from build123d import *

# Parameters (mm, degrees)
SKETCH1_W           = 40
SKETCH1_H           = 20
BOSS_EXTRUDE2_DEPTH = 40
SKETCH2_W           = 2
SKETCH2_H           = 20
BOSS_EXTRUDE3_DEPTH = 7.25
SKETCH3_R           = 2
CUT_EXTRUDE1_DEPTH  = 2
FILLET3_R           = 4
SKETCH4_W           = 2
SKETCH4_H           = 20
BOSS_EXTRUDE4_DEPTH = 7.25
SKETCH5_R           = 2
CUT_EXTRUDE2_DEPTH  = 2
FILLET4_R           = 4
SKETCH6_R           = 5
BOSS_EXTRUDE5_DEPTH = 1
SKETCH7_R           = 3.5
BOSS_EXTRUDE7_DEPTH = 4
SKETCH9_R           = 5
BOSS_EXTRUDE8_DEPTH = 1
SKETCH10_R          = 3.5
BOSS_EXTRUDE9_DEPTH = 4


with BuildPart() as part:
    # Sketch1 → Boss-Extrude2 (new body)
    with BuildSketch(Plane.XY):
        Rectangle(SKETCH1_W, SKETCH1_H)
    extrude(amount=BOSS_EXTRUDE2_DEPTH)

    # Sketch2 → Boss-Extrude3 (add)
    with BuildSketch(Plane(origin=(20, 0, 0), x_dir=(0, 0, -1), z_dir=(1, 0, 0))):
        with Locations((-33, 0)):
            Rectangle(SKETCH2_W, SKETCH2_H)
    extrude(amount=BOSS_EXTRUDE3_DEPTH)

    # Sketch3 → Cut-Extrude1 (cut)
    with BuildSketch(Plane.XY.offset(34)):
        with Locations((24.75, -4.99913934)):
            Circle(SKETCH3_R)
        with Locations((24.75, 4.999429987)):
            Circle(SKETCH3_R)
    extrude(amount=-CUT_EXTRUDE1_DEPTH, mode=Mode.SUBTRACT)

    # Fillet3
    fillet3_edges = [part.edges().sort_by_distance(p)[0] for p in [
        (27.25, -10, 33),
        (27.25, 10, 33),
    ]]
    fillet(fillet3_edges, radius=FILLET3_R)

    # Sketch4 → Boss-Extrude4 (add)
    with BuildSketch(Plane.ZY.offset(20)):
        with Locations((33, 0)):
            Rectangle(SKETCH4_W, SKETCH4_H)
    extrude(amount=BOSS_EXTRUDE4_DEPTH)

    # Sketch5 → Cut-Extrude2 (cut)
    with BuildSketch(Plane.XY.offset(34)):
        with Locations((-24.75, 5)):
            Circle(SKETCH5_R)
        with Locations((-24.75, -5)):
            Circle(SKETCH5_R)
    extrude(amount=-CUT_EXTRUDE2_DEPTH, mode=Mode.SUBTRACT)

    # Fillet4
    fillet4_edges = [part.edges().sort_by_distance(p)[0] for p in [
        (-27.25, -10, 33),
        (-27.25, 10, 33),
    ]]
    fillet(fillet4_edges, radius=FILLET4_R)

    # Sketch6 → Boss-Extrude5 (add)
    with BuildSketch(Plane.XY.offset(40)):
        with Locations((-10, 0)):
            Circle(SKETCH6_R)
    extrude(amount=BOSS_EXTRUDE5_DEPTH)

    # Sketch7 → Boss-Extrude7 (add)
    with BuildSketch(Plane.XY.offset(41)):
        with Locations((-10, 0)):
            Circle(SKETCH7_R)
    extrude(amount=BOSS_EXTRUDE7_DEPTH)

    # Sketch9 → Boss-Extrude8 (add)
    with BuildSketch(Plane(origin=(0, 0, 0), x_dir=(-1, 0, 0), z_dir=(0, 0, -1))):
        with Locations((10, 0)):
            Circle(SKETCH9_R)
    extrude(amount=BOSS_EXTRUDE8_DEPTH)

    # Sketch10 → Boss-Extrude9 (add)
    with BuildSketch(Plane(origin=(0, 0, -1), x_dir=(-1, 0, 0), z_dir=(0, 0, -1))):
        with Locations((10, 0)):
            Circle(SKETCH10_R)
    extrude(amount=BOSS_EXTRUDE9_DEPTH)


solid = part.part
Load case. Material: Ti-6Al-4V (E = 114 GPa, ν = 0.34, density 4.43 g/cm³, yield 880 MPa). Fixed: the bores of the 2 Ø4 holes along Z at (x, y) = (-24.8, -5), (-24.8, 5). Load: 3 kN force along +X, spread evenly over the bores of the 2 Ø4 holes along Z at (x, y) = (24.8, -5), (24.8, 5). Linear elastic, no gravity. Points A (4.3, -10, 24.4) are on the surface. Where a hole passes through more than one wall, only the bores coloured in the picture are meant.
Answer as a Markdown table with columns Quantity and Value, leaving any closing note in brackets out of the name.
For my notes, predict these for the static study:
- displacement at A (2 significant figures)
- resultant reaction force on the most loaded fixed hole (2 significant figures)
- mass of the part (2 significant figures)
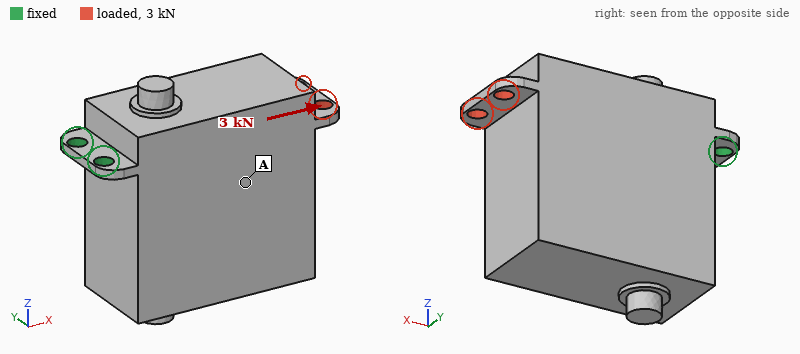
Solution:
| Quantity | Value |
|---|---|
| displacement at A | 5.4 µm |
| resultant reaction force on the most loaded fixed hole | 1.5 kN |
| mass of the part | 150 g |
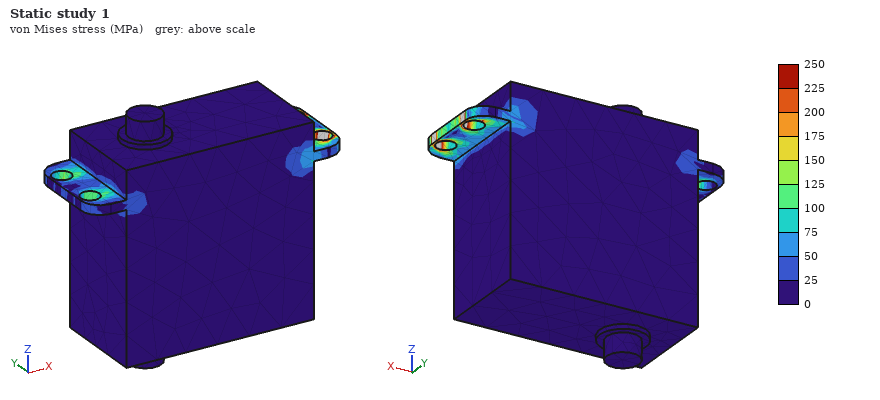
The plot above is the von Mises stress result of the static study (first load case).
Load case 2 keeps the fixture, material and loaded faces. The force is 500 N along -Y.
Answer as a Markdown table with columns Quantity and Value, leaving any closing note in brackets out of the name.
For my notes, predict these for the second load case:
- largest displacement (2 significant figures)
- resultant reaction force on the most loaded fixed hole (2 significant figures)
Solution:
| Quantity | Value |
|---|---|
| largest displacement | 73 µm |
| resultant reaction force on the most loaded fixed hole | 2.0 kN |
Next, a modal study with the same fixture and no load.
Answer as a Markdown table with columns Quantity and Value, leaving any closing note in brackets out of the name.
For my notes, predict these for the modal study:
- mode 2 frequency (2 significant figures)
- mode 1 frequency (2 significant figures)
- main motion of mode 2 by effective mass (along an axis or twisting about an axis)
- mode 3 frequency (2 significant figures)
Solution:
| Quantity | Value |
|---|---|
| mode 2 frequency | 1400 Hz |
| mode 1 frequency | 280 Hz |
| main motion of mode 2 by effective mass | along Y |
| mode 3 frequency | 3000 Hz |
